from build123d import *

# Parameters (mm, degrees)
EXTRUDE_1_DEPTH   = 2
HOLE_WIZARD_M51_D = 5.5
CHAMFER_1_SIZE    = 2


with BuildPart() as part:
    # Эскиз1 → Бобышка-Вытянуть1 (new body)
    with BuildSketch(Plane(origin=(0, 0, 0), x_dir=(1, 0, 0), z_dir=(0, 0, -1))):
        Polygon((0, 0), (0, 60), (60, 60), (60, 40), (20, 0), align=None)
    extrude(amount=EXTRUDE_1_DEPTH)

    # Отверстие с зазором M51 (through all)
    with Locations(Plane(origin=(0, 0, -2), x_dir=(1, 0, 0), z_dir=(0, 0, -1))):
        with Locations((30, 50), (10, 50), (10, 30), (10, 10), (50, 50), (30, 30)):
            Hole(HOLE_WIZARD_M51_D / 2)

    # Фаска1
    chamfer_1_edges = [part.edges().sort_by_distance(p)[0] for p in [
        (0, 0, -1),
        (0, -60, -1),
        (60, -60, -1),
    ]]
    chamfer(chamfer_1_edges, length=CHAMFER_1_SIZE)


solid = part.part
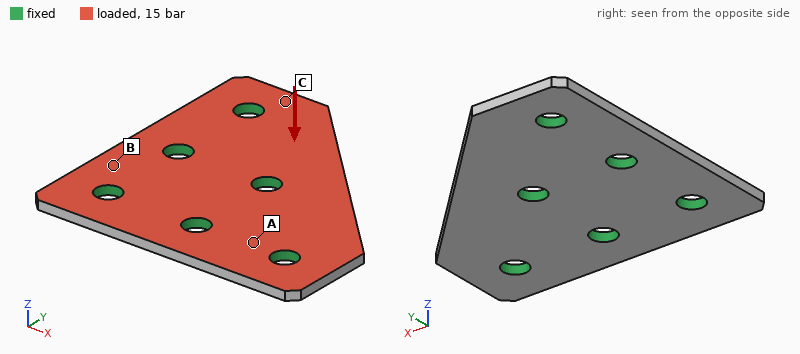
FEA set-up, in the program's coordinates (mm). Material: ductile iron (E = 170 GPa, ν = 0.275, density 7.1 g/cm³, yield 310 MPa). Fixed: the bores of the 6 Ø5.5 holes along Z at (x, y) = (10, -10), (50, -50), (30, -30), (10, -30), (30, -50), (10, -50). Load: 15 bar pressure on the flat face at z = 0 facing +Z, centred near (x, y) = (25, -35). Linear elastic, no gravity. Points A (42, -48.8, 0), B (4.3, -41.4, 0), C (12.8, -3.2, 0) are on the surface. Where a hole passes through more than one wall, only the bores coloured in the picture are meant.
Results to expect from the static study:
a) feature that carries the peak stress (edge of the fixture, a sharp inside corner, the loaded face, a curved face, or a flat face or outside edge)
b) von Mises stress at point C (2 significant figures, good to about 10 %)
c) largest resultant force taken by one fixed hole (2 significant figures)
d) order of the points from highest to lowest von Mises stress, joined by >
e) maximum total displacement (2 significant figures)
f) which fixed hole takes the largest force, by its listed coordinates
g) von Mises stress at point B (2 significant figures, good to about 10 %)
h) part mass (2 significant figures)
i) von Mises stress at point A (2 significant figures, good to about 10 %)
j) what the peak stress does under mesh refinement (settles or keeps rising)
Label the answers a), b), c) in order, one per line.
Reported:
a) edge of the fixture
b) 90 MPa
c) 920 N
d) C > A > B
e) 66 µm
f) (30, -30)
g) 28 MPa
h) 38 g
i) 53 MPa
j) keeps rising
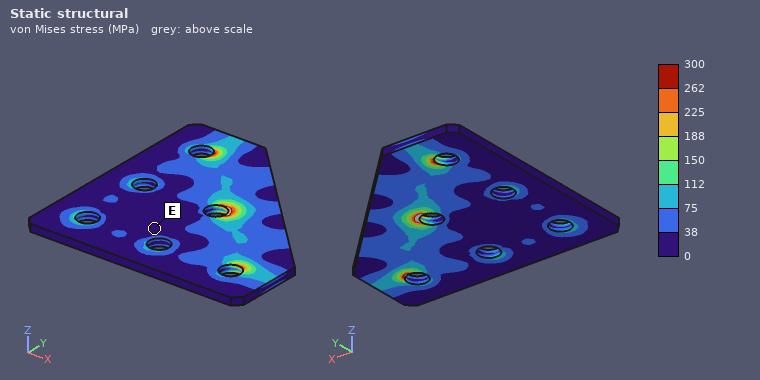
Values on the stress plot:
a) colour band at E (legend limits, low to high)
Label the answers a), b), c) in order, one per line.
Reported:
a) 0 to 38 MPa
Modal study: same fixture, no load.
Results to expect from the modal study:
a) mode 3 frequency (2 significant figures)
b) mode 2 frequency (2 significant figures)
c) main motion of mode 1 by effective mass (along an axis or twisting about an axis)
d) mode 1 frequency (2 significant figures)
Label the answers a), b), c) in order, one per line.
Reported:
a) 15 kHz
b) 9200 Hz
c) along Z
d) 8300 Hz
